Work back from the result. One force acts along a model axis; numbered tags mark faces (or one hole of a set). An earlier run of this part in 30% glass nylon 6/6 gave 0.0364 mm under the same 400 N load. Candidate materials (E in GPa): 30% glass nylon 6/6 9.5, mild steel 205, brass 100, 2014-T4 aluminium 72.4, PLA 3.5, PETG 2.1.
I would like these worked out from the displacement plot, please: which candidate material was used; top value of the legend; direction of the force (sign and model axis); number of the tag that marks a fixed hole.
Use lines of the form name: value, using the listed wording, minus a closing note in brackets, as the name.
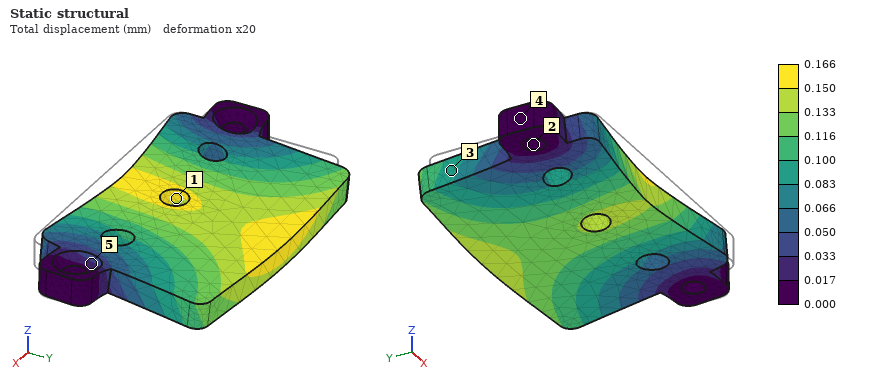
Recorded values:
which candidate material was used: PETG
top value of the legend: 0.166 mm
direction of the force: +Y
number of the tag that marks a fixed hole: 2
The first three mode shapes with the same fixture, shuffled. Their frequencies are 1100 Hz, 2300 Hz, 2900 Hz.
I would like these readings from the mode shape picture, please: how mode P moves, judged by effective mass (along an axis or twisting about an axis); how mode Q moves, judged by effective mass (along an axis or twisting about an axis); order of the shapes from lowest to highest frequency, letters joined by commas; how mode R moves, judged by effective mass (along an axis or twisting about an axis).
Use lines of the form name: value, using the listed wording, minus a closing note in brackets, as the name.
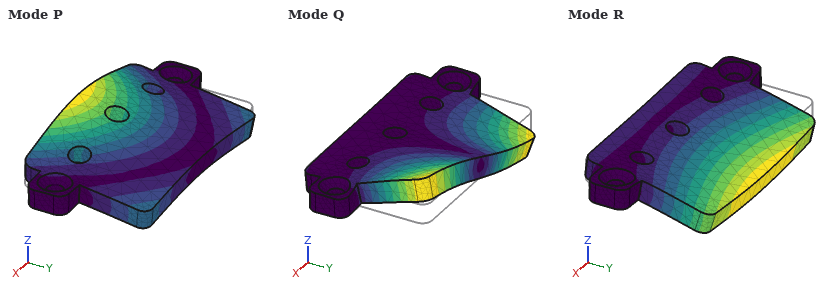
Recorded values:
how mode P moves, judged by effective mass: along Z
how mode Q moves, judged by effective mass: twisting about Y
order of the shapes from lowest to highest frequency, letters joined by commas: R, P, Q
how mode R moves, judged by effective mass: along Z
